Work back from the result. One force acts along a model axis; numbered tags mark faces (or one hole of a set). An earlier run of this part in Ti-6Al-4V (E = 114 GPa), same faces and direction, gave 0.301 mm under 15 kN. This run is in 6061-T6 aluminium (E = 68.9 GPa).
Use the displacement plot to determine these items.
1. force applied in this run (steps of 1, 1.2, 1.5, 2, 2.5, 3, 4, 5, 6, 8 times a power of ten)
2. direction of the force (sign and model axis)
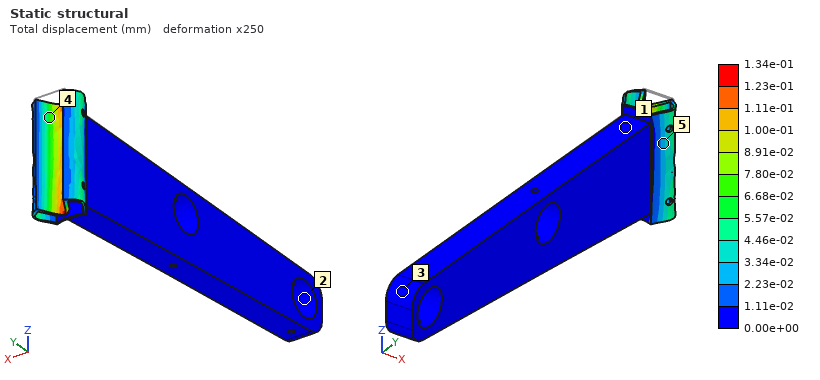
4 kN
-Y
